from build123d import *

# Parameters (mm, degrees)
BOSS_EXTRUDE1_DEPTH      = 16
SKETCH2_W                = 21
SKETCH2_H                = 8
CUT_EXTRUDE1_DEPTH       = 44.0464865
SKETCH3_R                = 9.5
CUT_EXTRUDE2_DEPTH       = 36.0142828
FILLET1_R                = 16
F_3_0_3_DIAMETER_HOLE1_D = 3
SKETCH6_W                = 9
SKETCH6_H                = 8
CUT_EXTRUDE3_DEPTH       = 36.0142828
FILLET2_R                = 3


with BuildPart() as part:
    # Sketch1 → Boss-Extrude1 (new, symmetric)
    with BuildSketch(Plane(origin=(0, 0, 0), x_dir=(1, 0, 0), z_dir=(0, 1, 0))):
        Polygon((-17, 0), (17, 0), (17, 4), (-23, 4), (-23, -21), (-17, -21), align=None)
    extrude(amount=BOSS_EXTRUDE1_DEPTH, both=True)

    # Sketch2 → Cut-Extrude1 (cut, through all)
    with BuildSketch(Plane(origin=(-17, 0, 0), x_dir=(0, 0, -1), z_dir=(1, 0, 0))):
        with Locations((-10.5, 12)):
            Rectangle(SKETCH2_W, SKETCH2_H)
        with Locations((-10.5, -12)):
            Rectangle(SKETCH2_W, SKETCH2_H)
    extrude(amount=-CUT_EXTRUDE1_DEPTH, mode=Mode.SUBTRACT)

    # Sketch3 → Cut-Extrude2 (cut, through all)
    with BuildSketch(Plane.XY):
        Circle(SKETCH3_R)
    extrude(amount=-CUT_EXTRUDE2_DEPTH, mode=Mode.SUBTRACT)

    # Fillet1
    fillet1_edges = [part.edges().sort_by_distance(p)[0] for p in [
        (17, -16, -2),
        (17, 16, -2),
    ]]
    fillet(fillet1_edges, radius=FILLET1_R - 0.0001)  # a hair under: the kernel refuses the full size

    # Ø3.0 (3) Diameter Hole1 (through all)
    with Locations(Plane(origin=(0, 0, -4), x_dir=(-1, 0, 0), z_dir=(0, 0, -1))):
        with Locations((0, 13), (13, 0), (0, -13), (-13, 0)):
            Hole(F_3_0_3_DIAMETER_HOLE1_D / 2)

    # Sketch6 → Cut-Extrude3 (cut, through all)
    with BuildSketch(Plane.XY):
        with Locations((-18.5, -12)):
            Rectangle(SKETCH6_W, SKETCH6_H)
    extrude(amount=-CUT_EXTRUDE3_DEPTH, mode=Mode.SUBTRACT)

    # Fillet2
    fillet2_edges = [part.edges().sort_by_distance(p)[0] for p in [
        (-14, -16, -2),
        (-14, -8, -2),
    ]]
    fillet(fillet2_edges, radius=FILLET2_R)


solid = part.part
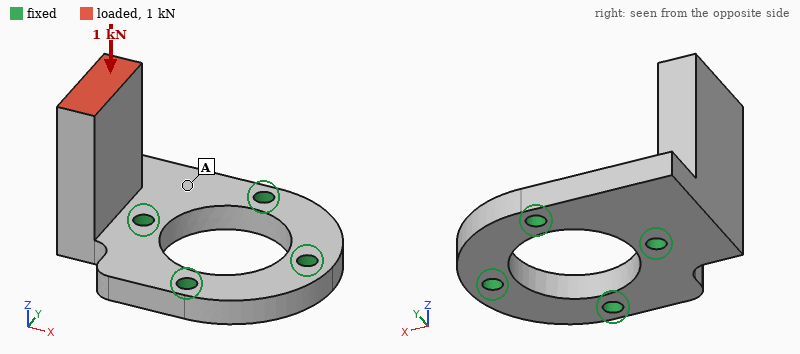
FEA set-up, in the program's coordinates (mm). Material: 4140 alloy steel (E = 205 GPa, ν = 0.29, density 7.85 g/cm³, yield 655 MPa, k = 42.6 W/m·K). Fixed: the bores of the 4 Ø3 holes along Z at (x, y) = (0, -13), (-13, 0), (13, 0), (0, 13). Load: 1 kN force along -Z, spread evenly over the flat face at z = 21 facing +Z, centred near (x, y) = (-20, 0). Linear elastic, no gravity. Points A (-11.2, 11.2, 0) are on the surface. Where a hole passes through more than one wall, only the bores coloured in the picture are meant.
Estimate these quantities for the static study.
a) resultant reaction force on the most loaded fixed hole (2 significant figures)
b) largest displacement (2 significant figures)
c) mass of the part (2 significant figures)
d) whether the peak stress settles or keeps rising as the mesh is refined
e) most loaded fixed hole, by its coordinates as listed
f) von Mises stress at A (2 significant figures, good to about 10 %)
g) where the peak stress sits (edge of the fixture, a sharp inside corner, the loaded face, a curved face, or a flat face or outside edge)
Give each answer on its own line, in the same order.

1.1 kN
33 µm
41 g
keeps rising
(-13, 0)
28 MPa
edge of the fixture
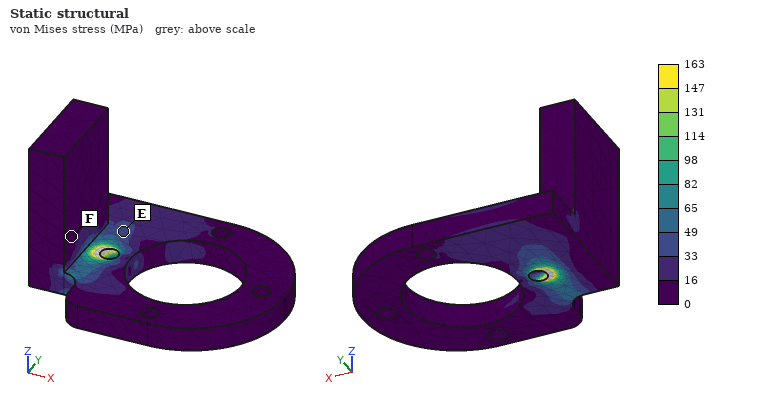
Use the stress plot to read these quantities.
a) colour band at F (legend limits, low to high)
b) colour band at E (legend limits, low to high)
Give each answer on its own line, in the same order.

0 to 16 MPa
33 to 49 MPa
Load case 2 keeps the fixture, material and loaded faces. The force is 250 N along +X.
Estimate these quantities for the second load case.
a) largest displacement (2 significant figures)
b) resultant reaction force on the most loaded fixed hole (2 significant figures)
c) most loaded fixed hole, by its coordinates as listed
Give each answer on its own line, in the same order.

55 µm
260 N
(-13, 0)
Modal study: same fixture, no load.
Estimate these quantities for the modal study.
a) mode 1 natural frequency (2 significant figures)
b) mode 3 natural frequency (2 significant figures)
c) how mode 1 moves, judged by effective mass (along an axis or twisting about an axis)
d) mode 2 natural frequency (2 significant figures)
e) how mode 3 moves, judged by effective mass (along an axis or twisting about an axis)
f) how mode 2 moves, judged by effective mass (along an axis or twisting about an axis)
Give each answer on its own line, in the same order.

4500 Hz
18 kHz
along X
6200 Hz
along Z
along Y
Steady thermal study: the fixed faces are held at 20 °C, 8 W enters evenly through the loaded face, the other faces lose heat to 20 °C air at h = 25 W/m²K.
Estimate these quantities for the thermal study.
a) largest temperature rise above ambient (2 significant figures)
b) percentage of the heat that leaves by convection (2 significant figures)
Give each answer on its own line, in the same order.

55 K
13 %
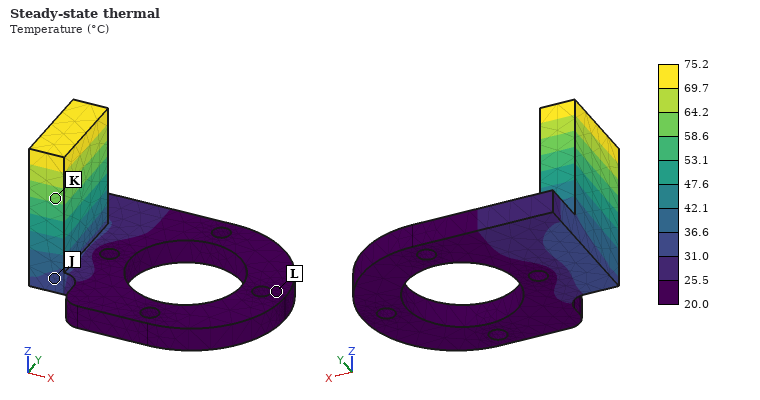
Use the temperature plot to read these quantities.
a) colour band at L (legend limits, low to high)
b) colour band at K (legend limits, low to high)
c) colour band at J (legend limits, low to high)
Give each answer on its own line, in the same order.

20.0 to 25.5 °C
58.6 to 64.2 °C
31.0 to 36.6 °C
